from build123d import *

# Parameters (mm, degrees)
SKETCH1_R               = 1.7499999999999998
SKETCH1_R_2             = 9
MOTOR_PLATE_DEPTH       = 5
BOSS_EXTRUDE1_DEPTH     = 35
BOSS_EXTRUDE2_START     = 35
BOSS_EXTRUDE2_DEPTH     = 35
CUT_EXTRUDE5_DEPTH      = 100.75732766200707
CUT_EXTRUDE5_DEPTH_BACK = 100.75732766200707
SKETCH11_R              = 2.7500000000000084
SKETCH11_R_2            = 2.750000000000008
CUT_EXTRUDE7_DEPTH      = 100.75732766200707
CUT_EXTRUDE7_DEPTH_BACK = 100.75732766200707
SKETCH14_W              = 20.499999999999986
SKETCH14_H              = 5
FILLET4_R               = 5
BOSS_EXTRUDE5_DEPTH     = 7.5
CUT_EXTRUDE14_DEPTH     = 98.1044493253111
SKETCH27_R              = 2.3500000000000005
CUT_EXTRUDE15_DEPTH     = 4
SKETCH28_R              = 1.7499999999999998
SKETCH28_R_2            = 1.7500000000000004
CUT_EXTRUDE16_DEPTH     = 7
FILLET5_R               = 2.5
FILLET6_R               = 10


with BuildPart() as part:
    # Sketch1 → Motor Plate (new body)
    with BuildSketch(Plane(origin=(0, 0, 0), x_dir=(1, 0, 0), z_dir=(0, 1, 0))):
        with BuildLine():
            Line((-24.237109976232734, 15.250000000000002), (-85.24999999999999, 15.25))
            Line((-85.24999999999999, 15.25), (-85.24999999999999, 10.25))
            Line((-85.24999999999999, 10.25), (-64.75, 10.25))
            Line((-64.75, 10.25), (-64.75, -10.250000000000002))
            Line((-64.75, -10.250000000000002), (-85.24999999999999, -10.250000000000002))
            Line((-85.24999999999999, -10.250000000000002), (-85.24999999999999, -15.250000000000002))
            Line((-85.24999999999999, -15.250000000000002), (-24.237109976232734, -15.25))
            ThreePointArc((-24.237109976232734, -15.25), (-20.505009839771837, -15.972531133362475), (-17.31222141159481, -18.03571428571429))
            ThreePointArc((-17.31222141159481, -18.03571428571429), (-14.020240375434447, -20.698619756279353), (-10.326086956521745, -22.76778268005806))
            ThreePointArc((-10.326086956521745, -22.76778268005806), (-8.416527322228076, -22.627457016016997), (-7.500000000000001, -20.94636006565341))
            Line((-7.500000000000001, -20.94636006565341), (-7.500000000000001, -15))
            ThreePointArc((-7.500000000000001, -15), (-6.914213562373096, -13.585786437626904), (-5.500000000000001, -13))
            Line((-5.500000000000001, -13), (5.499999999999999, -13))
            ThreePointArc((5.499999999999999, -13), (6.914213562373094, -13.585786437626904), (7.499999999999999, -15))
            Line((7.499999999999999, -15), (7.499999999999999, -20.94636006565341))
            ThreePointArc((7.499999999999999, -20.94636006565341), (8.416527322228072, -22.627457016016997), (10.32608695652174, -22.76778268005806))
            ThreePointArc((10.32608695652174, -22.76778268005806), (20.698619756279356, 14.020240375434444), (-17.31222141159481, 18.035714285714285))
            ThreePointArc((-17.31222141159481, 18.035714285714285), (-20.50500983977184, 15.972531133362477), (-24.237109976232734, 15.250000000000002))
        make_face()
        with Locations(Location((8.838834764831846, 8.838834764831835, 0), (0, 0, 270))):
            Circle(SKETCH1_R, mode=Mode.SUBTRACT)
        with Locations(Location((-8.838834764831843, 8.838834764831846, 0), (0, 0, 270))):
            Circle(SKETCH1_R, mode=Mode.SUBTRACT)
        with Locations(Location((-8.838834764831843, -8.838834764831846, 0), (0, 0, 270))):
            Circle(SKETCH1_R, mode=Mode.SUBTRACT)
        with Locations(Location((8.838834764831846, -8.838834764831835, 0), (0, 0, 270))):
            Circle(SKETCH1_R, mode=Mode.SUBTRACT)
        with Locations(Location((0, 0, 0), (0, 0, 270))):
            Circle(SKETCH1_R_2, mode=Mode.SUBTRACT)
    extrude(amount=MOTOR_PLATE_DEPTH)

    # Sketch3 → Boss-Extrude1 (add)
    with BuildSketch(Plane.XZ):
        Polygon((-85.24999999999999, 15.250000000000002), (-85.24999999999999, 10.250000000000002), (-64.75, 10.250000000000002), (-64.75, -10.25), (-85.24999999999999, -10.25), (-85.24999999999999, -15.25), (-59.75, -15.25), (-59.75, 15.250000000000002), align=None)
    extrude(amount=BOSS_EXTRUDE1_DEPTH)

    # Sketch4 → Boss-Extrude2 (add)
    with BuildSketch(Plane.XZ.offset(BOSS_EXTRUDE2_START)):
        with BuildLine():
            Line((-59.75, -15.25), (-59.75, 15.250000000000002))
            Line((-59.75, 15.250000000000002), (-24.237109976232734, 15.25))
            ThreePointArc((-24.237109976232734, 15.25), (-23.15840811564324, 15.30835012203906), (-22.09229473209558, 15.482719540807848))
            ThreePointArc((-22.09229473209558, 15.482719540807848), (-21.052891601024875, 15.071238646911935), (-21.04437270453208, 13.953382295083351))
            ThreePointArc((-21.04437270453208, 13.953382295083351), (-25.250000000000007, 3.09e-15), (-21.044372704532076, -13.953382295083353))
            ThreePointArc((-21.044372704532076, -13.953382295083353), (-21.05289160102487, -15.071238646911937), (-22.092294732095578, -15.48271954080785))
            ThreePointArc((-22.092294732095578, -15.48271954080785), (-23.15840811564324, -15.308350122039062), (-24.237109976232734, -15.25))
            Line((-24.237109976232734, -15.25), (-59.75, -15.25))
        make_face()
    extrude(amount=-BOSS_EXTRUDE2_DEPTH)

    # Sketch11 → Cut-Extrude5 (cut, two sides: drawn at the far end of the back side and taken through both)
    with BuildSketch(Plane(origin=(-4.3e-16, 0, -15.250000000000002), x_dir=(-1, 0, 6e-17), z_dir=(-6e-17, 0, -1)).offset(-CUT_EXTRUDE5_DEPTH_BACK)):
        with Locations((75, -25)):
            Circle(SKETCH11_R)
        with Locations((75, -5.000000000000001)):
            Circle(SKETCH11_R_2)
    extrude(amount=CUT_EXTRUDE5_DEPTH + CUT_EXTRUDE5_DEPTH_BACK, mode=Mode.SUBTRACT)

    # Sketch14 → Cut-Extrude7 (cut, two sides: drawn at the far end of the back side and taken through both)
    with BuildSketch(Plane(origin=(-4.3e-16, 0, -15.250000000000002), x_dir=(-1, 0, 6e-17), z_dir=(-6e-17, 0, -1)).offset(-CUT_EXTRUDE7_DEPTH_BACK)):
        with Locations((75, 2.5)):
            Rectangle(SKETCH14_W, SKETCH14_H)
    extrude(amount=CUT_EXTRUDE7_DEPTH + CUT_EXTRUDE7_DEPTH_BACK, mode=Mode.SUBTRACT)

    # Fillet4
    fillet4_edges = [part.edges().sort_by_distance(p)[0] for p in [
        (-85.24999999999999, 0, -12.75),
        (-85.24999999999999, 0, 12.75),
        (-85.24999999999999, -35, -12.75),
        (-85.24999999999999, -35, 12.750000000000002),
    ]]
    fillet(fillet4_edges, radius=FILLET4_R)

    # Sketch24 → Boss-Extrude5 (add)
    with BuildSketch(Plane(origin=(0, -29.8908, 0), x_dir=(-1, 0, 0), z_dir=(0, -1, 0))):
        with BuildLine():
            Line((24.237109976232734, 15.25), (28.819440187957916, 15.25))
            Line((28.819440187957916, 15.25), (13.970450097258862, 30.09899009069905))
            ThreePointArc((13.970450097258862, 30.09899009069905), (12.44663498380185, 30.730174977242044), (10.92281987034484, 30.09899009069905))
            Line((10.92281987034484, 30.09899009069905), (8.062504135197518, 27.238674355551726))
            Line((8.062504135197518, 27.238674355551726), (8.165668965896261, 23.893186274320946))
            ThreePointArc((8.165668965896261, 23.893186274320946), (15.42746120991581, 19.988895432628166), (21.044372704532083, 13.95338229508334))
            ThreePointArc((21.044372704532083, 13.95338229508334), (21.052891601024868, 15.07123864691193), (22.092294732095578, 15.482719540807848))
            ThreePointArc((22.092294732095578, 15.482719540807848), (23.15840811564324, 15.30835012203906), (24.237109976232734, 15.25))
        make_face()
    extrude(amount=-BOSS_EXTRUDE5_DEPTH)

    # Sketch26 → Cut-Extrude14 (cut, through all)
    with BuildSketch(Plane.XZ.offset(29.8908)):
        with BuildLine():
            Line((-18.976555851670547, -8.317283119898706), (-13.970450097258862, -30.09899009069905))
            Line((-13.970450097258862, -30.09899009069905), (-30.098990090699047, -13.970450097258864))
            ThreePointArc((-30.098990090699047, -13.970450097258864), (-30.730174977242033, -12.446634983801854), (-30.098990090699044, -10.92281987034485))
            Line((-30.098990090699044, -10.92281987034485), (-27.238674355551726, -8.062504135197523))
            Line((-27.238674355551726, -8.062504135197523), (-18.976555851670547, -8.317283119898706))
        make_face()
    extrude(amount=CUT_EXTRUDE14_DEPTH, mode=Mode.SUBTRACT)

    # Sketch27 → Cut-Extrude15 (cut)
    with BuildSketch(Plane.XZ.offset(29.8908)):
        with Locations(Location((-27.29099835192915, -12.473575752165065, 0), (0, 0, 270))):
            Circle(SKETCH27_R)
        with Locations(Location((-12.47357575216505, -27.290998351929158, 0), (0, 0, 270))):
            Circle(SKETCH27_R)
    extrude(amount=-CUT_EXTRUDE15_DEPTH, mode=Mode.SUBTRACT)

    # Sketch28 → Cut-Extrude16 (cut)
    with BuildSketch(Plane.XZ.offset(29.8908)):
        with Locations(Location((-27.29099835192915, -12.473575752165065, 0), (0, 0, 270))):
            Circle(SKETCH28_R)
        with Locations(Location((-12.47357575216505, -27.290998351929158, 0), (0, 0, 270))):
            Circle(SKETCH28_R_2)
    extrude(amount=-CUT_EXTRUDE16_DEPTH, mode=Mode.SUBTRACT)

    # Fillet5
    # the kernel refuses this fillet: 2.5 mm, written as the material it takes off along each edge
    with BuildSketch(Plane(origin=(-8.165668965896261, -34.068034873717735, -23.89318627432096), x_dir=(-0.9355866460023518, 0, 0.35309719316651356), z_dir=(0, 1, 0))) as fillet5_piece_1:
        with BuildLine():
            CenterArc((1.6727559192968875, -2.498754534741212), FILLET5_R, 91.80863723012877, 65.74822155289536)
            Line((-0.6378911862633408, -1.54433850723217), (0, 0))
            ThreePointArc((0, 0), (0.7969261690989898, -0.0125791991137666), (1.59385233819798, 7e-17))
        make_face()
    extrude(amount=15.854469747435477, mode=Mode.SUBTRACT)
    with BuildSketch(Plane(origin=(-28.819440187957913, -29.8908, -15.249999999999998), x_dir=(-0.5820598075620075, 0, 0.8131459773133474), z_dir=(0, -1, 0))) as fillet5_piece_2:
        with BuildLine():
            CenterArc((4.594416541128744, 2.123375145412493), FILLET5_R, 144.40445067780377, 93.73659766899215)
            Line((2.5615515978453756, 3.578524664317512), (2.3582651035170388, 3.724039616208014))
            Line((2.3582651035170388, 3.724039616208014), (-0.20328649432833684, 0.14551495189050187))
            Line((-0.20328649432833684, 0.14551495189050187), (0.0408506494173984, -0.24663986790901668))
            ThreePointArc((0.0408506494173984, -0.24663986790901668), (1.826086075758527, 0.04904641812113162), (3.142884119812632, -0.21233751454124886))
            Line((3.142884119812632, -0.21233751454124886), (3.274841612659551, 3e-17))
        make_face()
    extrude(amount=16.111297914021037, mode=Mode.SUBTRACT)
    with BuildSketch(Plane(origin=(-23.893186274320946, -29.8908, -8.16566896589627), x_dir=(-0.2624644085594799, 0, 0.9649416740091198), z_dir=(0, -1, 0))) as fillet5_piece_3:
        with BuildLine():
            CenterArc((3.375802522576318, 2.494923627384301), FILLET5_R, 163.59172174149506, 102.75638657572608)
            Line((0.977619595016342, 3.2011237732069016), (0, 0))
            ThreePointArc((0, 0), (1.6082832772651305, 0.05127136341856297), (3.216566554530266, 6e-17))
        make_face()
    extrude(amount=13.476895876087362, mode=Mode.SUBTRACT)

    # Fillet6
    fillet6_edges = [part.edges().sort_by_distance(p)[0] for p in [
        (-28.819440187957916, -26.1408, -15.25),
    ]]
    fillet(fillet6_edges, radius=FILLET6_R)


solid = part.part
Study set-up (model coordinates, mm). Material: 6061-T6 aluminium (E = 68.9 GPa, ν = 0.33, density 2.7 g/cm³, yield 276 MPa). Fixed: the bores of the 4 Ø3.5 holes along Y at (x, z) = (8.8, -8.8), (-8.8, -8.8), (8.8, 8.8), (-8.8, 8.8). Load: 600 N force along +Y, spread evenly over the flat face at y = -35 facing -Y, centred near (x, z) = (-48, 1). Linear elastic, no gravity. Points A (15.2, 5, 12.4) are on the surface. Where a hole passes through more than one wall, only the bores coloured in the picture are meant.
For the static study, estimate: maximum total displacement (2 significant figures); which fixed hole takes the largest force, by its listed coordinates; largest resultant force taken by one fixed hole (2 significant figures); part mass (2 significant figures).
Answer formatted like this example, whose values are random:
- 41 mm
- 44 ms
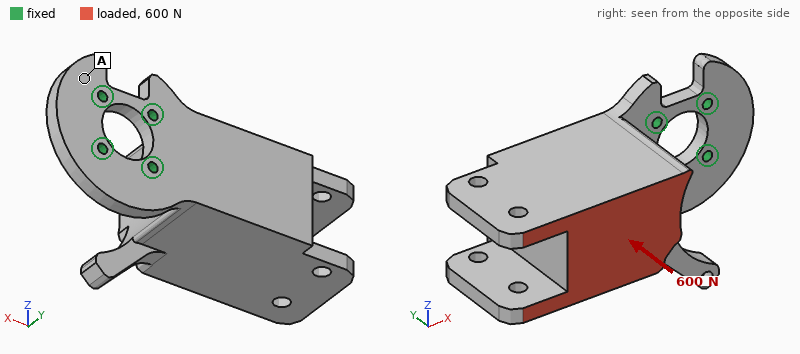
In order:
- 1.0 mm
- (-8.8, -8.8)
- 450 N
- 170 g
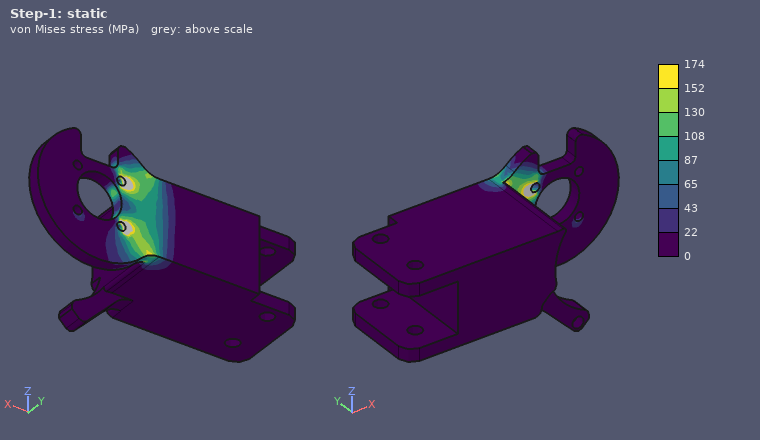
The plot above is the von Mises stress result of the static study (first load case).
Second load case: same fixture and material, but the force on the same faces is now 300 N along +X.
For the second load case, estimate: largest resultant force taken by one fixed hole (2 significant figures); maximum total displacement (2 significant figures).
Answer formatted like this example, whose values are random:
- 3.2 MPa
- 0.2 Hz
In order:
- 160 N
- 0.62 mm
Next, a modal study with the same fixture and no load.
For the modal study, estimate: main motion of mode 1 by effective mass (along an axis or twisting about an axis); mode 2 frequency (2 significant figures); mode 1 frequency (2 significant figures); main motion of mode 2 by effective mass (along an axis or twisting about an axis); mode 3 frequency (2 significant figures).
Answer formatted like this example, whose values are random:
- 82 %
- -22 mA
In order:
- along Y
- 1300 Hz
- 380 Hz
- along Z
- 2900 Hz
